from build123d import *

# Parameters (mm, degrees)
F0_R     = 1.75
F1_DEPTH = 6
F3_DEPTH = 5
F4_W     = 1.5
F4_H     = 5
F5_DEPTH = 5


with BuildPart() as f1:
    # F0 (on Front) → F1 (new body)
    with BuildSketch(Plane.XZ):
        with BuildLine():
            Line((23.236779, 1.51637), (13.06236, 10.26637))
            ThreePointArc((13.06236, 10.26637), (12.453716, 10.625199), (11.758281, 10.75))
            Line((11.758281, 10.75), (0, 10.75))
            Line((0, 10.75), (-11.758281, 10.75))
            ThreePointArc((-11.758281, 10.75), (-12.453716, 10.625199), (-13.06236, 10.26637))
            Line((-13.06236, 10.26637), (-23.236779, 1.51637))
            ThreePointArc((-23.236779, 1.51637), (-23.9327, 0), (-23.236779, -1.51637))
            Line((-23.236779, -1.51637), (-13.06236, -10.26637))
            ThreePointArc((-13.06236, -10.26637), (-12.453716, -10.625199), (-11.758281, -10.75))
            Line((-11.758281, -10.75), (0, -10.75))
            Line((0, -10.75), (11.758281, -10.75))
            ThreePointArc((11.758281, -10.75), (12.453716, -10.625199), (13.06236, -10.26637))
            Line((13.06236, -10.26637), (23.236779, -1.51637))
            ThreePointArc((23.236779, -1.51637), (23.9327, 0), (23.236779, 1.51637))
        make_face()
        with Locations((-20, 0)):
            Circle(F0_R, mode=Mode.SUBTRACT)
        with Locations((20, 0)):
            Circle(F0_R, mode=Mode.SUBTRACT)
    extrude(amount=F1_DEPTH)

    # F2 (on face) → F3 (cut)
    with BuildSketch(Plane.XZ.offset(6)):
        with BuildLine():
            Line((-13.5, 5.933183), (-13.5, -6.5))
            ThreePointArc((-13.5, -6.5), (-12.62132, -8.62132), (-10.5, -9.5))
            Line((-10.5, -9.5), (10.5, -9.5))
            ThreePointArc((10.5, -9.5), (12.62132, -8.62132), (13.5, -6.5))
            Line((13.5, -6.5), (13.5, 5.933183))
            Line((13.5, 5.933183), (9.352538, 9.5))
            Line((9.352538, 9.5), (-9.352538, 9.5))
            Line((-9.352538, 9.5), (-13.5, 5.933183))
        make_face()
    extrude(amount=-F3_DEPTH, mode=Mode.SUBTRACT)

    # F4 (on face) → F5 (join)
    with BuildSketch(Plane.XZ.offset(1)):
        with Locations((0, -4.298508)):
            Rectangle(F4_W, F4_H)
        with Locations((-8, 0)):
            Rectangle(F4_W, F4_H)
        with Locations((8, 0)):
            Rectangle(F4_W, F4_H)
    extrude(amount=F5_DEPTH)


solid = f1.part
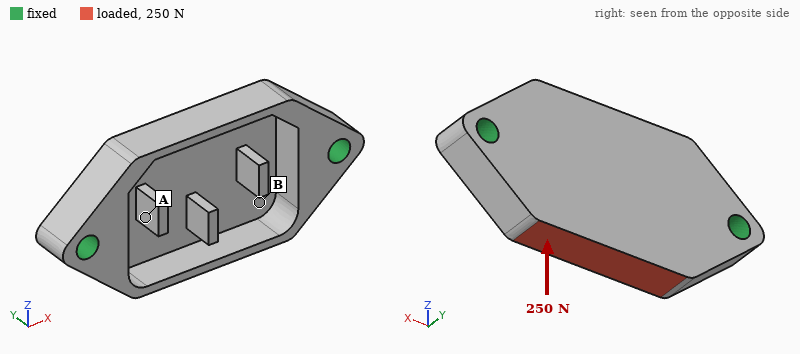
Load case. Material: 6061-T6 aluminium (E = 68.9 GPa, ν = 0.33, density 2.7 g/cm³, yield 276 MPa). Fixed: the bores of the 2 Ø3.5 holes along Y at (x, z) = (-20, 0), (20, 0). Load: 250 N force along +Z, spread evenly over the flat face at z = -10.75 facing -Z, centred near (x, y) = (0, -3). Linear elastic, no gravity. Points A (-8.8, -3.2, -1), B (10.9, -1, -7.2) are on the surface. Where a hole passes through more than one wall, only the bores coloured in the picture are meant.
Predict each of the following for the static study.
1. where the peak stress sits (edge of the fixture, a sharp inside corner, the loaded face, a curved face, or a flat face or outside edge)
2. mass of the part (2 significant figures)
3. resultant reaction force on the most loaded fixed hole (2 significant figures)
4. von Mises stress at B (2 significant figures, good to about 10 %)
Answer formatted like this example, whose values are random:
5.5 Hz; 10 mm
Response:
a curved face; 6.3 g; 140 N; 20 MPa
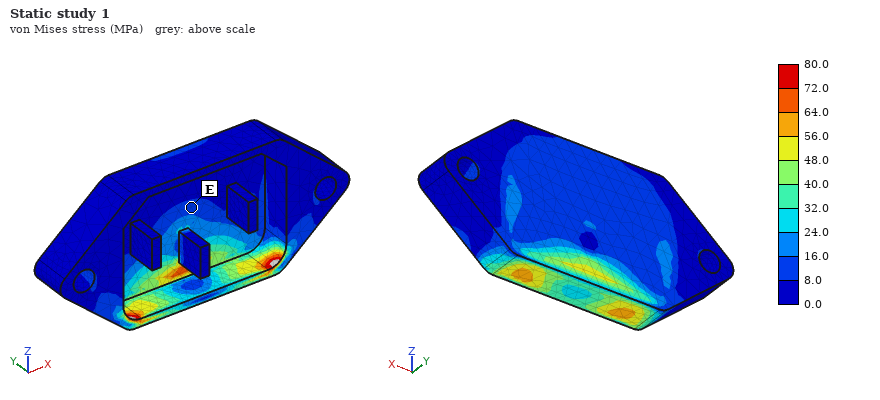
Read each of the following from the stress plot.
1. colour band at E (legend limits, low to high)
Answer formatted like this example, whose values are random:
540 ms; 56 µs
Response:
8.0 to 16.0 MPa
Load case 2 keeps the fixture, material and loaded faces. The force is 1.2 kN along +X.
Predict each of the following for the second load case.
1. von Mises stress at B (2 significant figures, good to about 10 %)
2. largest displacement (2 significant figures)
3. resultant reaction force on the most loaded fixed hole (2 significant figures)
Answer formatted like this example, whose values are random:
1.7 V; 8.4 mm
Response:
54 MPa; 27 µm; 670 N
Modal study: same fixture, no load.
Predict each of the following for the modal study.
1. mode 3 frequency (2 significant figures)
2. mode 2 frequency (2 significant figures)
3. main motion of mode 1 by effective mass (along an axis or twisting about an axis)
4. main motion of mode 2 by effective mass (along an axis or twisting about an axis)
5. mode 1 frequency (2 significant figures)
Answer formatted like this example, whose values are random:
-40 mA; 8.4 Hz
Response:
19 kHz; 16 kHz; along Y; twisting about X; 10 kHz
